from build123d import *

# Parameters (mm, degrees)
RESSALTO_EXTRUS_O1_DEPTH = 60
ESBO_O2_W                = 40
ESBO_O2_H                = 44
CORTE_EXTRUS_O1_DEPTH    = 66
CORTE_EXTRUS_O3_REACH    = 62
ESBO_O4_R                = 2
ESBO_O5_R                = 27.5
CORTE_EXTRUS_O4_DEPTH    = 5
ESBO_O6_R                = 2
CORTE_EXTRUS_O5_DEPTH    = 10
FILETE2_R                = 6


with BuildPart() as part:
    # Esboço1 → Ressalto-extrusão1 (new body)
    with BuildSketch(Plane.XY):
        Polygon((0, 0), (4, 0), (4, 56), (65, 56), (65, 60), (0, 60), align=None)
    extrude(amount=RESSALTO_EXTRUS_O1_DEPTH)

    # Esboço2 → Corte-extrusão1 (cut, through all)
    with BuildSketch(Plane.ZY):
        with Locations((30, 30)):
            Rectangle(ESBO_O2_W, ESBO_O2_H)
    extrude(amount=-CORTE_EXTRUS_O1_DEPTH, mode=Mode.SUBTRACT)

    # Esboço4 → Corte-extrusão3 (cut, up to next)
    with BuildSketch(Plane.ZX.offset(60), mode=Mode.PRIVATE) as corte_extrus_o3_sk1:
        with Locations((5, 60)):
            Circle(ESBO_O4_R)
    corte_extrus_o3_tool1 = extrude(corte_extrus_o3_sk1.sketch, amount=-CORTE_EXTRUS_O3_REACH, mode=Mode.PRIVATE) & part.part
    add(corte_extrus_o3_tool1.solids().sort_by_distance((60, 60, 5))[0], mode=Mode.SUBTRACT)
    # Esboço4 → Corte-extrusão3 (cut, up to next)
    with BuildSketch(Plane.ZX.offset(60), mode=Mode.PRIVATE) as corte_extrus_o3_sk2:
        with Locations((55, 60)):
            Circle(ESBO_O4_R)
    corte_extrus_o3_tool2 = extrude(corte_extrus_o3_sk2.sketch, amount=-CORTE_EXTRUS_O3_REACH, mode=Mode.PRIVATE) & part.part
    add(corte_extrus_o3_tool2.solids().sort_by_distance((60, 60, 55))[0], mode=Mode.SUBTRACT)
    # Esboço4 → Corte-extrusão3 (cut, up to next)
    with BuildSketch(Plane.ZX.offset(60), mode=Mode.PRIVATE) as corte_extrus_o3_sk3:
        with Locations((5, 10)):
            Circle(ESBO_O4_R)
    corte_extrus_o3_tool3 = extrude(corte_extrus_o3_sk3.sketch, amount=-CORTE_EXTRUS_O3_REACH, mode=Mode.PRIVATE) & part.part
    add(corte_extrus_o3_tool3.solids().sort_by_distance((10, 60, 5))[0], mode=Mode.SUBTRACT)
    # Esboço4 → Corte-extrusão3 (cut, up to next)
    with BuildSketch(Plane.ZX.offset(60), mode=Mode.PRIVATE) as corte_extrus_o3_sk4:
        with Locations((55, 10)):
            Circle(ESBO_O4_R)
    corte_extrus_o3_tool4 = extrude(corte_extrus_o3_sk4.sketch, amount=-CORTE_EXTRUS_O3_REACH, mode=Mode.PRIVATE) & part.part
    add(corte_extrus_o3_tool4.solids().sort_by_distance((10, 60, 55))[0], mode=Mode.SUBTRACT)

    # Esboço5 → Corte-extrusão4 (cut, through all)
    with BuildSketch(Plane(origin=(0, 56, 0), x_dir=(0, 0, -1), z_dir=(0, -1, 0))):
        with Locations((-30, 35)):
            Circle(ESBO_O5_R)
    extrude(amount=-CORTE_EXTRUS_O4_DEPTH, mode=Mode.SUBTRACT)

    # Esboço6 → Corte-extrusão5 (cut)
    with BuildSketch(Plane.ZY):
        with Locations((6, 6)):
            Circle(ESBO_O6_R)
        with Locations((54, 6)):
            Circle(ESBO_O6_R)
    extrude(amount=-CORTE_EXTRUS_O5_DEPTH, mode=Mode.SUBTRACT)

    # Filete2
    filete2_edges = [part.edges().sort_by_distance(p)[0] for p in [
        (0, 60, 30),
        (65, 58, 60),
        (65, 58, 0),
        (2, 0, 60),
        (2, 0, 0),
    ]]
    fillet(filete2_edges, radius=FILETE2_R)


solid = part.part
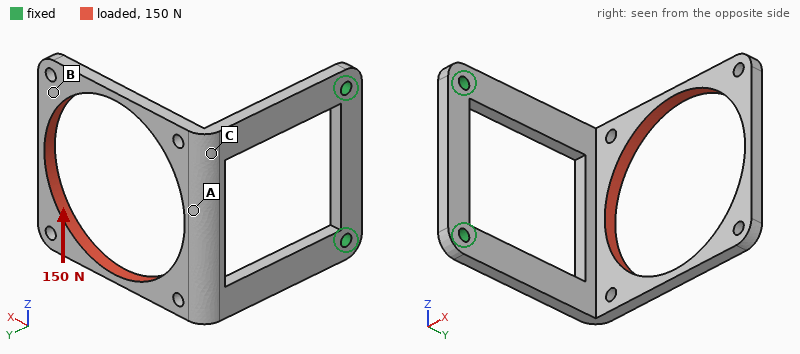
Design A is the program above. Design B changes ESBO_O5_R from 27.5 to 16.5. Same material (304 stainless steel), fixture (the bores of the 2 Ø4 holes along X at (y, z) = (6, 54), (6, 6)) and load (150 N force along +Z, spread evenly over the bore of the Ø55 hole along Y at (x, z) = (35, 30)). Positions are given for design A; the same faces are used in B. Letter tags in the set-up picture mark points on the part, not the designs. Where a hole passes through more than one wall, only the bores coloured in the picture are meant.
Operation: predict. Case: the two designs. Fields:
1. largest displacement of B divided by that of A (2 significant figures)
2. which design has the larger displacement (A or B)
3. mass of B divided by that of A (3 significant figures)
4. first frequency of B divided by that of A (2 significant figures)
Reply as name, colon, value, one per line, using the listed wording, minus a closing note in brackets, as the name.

largest displacement of B divided by that of A: 0.83
which design has the larger displacement: A
mass of B divided by that of A: 1.52
first frequency of B divided by that of A: 0.74
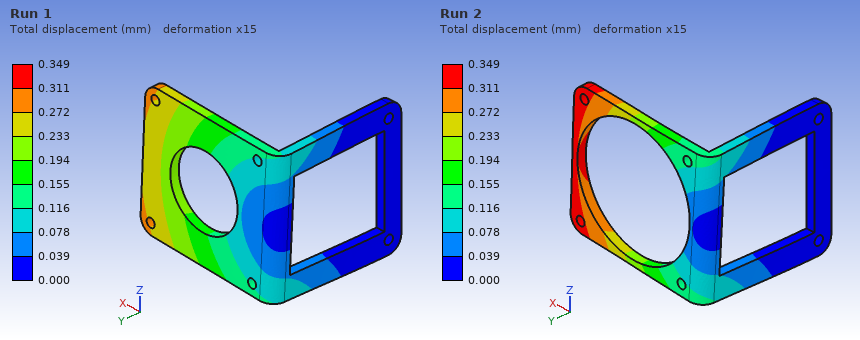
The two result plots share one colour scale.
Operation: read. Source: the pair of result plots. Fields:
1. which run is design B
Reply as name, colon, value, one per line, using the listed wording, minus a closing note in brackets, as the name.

which run is design B: Run 1
